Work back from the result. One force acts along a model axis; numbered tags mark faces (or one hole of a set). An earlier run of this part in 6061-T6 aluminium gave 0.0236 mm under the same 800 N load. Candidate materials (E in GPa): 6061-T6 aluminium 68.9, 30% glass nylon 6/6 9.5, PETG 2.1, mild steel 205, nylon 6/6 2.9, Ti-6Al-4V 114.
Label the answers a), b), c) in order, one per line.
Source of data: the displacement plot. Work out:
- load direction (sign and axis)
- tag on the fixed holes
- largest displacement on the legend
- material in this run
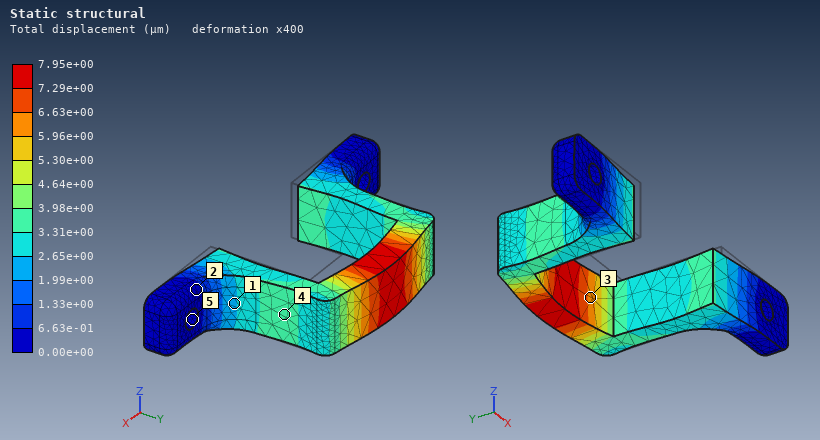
a) +Y
b) 5
c) 7.95e+00 µm
d) mild steel
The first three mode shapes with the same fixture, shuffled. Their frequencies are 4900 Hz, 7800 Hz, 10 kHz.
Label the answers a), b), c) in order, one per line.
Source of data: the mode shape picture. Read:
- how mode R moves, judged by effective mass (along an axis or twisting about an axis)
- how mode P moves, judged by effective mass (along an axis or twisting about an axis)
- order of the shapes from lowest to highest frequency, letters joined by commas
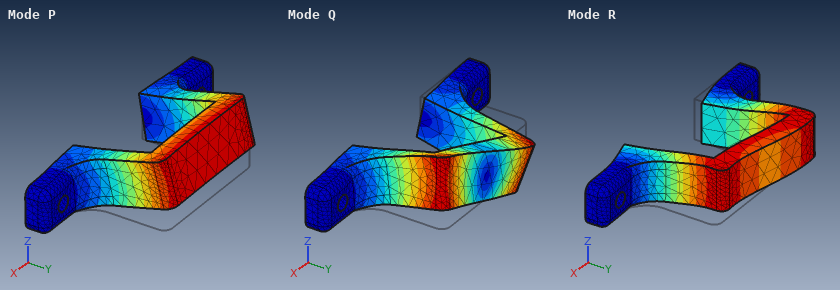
a) along X
b) along Z
c) P, R, Q
